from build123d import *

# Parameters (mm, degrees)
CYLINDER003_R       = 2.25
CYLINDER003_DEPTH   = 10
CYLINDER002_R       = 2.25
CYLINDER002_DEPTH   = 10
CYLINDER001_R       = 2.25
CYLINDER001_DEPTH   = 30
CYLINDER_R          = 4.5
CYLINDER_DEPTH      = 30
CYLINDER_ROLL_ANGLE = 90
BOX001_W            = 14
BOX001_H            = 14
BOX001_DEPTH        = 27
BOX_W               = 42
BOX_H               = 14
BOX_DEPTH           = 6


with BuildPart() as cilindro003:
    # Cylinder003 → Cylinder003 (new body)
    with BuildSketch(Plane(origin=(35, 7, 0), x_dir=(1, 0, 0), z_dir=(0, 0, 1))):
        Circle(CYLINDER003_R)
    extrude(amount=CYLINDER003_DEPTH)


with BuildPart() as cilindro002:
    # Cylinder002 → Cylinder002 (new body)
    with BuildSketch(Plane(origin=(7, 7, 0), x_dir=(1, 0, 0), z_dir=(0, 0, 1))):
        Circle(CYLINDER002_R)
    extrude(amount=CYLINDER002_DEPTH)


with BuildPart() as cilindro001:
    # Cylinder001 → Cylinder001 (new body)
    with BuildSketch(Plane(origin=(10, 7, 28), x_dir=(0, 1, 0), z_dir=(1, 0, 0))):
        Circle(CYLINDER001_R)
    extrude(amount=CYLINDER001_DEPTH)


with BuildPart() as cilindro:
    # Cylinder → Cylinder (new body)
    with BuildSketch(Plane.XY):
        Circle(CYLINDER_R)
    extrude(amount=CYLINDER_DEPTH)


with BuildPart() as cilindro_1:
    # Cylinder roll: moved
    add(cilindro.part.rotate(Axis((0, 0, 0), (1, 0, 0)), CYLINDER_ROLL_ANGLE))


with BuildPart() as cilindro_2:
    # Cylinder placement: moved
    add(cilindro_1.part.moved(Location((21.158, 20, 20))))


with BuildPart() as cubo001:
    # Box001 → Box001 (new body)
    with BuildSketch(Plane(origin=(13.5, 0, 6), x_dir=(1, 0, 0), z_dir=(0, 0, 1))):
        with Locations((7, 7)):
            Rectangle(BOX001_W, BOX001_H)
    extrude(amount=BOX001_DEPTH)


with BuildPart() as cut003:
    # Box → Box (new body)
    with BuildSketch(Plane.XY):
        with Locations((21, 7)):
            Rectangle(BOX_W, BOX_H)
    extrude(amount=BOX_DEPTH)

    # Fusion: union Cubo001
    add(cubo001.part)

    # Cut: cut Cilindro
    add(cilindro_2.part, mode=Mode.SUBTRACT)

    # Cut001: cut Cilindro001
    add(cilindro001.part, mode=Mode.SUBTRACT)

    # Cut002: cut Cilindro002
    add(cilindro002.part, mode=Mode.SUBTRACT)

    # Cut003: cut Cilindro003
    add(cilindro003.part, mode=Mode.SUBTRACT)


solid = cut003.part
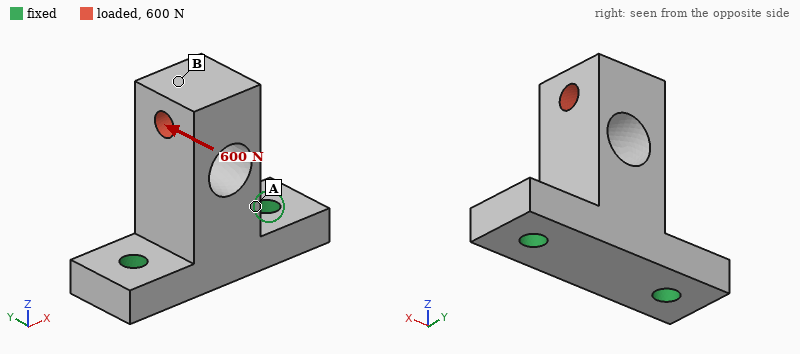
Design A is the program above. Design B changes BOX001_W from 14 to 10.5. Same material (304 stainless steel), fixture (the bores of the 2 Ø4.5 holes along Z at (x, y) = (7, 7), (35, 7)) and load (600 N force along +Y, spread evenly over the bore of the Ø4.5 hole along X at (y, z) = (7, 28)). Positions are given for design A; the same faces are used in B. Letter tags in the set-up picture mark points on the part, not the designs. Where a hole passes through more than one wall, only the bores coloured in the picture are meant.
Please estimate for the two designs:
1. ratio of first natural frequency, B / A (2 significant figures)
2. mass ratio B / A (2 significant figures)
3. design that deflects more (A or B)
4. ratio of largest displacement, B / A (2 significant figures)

1.0
0.83
B
1.5
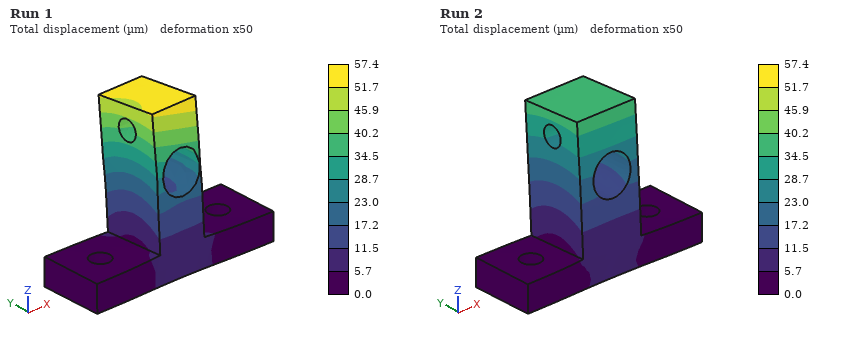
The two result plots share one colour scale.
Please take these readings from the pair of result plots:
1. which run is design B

Run 1
